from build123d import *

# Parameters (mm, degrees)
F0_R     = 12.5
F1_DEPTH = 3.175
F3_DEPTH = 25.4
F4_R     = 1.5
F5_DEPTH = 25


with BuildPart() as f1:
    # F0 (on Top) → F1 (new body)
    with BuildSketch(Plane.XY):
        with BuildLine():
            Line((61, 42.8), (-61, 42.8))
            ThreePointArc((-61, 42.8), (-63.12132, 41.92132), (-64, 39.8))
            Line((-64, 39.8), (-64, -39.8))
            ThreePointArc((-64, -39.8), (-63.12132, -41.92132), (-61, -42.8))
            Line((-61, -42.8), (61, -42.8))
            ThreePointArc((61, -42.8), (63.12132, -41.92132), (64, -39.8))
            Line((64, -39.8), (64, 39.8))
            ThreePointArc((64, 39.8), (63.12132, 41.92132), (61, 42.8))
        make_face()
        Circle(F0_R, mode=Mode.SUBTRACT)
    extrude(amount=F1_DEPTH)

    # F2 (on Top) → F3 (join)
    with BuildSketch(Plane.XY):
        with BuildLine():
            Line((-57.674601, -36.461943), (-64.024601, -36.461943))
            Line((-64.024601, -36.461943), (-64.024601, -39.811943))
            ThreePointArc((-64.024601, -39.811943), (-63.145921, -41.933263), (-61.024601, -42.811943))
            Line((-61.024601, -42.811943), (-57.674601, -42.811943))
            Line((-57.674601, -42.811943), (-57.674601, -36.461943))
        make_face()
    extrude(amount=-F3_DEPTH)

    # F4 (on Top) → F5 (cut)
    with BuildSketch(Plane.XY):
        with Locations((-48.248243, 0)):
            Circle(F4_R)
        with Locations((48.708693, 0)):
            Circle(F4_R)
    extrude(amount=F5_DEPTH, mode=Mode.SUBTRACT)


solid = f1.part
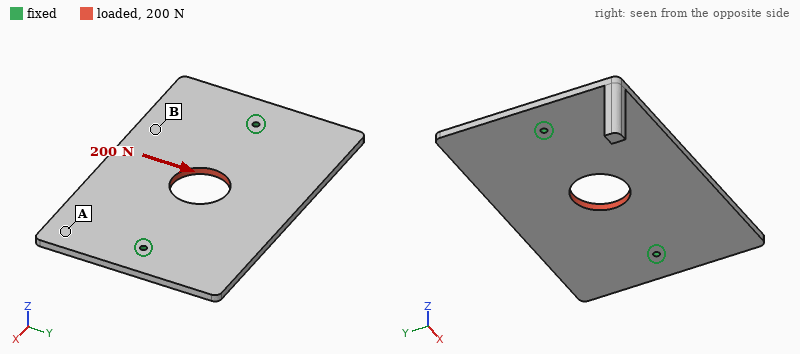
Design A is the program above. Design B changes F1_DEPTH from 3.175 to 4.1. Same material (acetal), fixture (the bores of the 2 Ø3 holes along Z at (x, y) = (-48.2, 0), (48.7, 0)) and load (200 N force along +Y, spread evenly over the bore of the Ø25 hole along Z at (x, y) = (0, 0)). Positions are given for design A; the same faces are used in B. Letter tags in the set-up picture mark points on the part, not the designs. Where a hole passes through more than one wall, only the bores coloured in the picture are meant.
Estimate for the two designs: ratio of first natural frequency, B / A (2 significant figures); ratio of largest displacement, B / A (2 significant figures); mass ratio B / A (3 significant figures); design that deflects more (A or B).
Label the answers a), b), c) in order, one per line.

a) 1.3
b) 0.77
c) 1.28
d) A
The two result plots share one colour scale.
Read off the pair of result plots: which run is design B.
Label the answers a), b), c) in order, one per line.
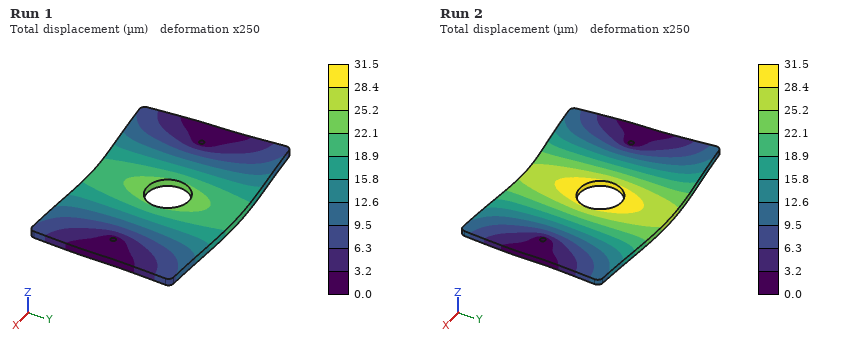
a) Run 1
